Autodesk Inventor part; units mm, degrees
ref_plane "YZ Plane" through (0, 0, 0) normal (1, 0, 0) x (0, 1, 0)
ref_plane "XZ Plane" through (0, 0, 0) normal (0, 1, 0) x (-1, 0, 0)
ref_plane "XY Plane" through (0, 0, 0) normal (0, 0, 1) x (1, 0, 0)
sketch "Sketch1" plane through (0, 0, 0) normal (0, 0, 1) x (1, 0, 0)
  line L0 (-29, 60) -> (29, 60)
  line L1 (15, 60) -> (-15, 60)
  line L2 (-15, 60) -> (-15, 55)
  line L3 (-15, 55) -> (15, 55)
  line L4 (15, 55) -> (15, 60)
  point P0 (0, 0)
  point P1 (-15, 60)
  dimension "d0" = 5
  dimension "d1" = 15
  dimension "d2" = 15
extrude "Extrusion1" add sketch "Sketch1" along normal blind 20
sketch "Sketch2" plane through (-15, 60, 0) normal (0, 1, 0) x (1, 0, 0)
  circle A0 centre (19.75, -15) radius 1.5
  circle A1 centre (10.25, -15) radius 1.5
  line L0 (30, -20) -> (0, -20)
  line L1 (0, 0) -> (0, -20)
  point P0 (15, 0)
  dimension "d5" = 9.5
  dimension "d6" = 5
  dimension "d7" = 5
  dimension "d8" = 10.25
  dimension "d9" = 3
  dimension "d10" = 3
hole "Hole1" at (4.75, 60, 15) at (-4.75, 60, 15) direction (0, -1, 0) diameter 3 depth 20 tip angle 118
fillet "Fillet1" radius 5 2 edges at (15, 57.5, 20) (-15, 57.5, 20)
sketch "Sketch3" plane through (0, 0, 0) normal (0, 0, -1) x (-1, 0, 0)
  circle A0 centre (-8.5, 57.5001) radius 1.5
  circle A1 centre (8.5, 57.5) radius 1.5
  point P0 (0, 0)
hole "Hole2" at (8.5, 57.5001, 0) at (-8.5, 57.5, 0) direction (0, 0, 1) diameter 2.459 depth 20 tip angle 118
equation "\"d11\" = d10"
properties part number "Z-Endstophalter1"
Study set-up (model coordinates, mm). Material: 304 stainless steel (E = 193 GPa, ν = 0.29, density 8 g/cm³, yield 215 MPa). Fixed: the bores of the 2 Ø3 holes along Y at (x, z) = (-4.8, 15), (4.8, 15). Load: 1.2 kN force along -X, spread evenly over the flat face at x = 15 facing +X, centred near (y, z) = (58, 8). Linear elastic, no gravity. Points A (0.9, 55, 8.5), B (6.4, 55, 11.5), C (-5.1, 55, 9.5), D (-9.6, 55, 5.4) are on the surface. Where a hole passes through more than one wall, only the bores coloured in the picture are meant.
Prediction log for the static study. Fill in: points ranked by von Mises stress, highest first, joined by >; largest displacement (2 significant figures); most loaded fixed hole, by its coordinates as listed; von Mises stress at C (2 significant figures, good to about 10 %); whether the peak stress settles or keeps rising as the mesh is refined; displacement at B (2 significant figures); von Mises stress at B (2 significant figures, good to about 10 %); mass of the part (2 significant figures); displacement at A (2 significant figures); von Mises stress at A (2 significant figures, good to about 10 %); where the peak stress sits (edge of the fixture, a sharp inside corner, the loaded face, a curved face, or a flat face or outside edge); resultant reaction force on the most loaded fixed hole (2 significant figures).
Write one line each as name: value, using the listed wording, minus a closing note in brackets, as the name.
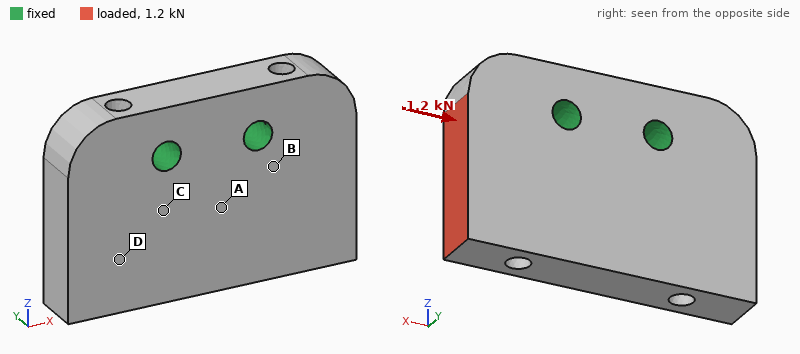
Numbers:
points ranked by von Mises stress, highest first, joined by >: B > A > C > D
largest displacement: 5.1 µm
most loaded fixed hole, by its coordinates as listed: (4.8, 15)
von Mises stress at C: 15 MPa
whether the peak stress settles or keeps rising as the mesh is refined: keeps rising
displacement at B: 1.1 µm
von Mises stress at B: 34 MPa
mass of the part: 21 g
displacement at A: 1.3 µm
von Mises stress at A: 23 MPa
where the peak stress sits: edge of the fixture
resultant reaction force on the most loaded fixed hole: 1.0 kN
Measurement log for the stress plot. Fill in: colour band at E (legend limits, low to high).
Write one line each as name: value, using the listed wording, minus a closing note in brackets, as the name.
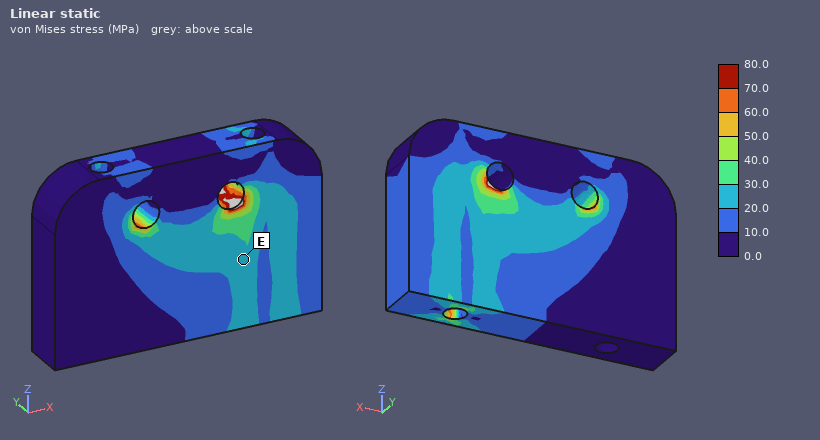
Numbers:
colour band at E: 20.0 to 30.0 MPa
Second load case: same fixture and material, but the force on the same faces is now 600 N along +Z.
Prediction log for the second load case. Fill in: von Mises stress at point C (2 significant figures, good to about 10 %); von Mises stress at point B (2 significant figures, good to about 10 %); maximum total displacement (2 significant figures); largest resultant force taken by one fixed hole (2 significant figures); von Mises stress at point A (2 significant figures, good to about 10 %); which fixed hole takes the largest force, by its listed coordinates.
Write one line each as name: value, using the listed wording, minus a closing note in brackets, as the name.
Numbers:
von Mises stress at point C: 10 MPa
von Mises stress at point B: 23 MPa
maximum total displacement: 4.9 µm
largest resultant force taken by one fixed hole: 1.0 kN
von Mises stress at point A: 12 MPa
which fixed hole takes the largest force, by its listed coordinates: (4.8, 15)
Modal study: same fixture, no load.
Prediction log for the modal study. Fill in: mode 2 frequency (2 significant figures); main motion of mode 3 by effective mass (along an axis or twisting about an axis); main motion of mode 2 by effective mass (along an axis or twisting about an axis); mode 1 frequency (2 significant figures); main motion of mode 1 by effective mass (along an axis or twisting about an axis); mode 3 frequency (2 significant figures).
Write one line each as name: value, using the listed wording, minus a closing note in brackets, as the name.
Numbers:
mode 2 frequency: 17 kHz
main motion of mode 3 by effective mass: along X
main motion of mode 2 by effective mass: twisting about Z
mode 1 frequency: 15 kHz
main motion of mode 1 by effective mass: along Y
mode 3 frequency: 24 kHz
